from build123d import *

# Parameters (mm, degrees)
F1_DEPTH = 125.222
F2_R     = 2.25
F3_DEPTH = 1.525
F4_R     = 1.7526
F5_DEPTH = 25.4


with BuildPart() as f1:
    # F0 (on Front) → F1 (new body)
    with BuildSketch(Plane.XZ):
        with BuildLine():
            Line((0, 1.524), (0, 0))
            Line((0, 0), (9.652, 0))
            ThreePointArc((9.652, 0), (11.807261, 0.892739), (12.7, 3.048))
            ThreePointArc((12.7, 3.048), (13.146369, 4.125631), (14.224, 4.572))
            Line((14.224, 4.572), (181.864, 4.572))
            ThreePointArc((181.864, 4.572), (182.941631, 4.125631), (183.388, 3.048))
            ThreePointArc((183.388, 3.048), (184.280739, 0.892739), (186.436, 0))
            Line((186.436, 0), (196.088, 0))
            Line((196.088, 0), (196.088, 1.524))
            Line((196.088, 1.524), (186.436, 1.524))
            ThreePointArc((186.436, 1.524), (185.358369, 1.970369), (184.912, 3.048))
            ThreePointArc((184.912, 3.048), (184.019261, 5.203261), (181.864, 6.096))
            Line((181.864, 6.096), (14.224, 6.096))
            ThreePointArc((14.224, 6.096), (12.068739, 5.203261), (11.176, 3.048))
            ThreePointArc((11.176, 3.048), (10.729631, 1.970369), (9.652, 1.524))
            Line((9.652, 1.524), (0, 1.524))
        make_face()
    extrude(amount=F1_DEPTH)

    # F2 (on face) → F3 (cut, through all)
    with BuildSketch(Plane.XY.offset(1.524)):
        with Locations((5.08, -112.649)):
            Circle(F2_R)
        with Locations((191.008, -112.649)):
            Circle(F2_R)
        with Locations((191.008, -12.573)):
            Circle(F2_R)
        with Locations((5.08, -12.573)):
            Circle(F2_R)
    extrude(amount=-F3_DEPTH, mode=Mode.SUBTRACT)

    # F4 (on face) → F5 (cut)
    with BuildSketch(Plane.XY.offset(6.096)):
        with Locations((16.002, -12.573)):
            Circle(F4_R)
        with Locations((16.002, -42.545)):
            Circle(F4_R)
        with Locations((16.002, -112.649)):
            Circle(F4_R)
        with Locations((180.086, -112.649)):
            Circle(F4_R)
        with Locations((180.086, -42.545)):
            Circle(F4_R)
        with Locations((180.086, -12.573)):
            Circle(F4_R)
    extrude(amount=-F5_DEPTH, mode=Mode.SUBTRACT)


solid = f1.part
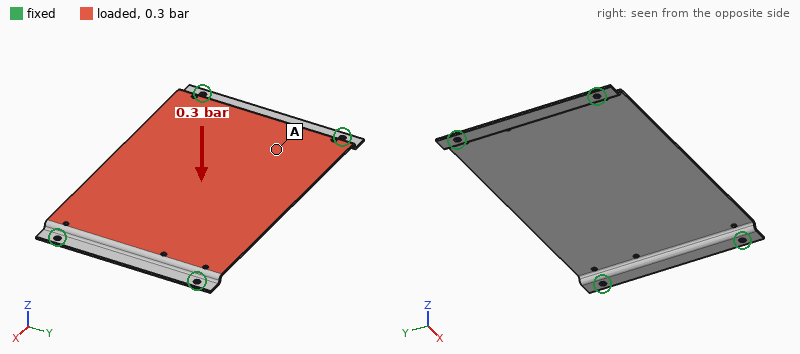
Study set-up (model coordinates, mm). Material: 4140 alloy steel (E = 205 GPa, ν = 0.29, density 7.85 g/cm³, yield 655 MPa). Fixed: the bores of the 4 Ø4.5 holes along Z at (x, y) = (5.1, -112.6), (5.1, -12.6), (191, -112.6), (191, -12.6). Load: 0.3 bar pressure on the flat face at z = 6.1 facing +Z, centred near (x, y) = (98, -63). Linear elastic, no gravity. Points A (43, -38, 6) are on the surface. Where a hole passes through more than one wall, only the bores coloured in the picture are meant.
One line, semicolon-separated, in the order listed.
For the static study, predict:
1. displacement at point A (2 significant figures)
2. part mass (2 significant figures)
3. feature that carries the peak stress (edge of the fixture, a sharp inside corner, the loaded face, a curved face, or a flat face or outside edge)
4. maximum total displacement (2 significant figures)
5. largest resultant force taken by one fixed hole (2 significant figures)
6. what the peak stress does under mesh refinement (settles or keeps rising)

0.54 mm; 300 g; a sharp inside corner; 1.4 mm; 1.1 kN; keeps rising
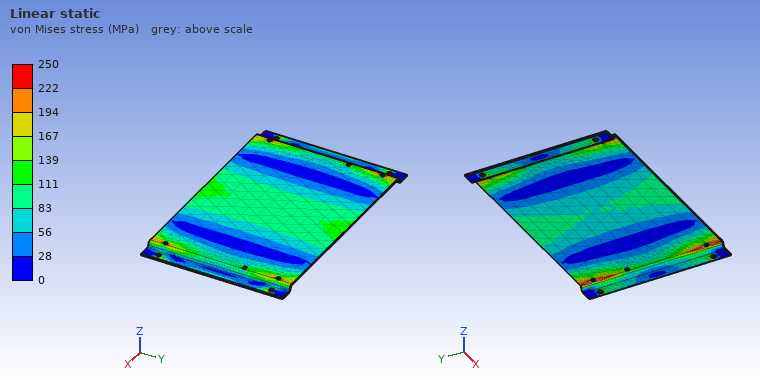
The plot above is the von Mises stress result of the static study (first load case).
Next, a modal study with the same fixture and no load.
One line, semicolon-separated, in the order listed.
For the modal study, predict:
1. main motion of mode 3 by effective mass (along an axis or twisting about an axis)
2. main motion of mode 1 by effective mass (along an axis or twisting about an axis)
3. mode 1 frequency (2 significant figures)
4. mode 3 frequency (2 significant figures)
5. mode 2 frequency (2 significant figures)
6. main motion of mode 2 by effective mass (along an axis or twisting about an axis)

twisting about Y; along Z; 250 Hz; 570 Hz; 360 Hz; twisting about X
